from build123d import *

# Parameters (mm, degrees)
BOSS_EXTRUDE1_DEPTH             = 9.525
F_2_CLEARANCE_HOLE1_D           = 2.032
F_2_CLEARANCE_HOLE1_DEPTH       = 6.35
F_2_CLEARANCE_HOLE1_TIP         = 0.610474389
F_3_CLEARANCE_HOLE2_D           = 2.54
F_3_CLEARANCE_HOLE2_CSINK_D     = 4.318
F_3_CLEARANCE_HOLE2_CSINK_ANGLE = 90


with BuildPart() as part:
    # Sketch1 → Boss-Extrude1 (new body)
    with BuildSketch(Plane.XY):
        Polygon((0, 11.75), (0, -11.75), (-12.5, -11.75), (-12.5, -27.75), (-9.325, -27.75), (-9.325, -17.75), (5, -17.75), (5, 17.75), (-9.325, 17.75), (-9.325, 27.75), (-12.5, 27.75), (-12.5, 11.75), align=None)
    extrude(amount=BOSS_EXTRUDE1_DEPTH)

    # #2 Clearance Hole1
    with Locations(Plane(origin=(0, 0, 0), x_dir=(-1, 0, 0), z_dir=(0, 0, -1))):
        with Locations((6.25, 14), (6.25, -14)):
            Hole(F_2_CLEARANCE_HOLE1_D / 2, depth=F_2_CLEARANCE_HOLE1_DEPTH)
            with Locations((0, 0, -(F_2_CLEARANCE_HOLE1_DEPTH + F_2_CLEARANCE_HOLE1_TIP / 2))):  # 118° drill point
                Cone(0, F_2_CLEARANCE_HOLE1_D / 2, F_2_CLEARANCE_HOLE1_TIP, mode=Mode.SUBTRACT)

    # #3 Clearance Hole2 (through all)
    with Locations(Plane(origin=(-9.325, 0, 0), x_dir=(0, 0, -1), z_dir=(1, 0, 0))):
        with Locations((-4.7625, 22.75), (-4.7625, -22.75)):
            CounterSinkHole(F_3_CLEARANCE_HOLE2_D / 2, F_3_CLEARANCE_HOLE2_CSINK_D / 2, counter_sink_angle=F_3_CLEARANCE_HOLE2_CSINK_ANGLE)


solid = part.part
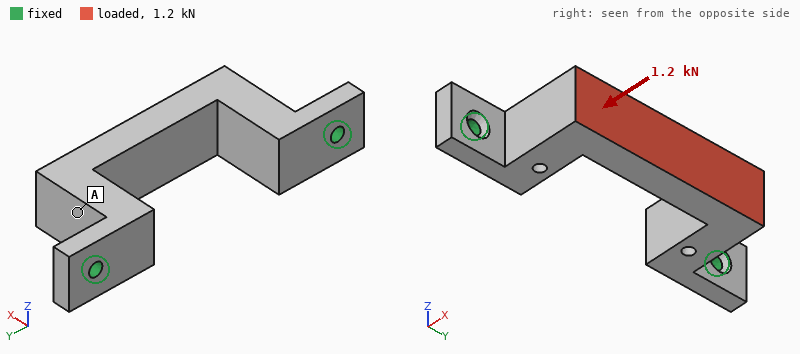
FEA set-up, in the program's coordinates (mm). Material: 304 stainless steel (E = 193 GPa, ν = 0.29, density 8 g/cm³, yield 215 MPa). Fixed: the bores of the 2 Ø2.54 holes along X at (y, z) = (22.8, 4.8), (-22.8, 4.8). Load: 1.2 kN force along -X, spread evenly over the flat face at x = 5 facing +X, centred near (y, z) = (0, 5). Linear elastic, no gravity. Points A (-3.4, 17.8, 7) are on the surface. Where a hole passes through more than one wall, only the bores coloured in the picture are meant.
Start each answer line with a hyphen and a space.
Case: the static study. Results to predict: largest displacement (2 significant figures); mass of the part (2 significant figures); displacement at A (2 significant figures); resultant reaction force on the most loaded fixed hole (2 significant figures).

- 11 µm
- 29 g
- 6.3 µm
- 710 N
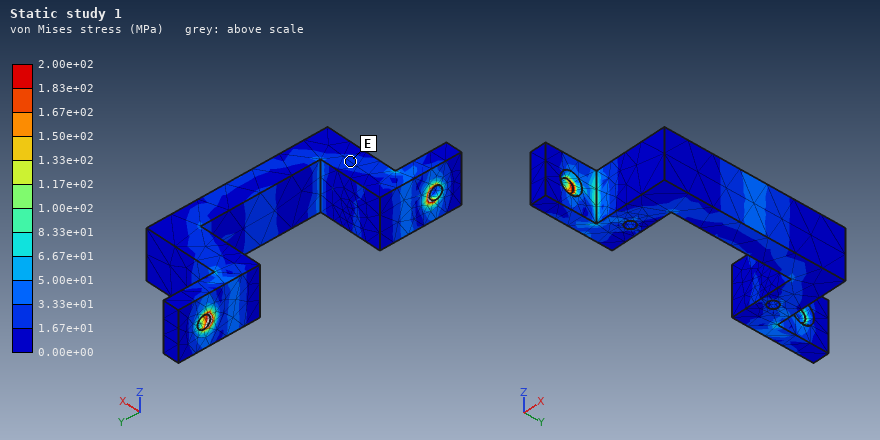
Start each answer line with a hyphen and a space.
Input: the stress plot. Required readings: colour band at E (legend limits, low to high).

- 1.67e+01 to 3.33e+01 MPa
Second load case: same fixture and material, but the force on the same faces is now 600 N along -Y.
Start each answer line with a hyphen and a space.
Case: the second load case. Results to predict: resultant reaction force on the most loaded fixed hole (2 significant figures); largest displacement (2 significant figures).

- 370 N
- 10 µm
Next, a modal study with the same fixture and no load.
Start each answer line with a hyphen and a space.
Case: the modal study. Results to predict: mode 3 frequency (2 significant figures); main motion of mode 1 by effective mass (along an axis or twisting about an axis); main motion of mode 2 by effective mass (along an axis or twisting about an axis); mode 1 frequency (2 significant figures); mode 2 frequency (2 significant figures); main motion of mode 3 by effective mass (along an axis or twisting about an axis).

- 10 kHz
- along Z
- along Y
- 3800 Hz
- 9400 Hz
- twisting about X
